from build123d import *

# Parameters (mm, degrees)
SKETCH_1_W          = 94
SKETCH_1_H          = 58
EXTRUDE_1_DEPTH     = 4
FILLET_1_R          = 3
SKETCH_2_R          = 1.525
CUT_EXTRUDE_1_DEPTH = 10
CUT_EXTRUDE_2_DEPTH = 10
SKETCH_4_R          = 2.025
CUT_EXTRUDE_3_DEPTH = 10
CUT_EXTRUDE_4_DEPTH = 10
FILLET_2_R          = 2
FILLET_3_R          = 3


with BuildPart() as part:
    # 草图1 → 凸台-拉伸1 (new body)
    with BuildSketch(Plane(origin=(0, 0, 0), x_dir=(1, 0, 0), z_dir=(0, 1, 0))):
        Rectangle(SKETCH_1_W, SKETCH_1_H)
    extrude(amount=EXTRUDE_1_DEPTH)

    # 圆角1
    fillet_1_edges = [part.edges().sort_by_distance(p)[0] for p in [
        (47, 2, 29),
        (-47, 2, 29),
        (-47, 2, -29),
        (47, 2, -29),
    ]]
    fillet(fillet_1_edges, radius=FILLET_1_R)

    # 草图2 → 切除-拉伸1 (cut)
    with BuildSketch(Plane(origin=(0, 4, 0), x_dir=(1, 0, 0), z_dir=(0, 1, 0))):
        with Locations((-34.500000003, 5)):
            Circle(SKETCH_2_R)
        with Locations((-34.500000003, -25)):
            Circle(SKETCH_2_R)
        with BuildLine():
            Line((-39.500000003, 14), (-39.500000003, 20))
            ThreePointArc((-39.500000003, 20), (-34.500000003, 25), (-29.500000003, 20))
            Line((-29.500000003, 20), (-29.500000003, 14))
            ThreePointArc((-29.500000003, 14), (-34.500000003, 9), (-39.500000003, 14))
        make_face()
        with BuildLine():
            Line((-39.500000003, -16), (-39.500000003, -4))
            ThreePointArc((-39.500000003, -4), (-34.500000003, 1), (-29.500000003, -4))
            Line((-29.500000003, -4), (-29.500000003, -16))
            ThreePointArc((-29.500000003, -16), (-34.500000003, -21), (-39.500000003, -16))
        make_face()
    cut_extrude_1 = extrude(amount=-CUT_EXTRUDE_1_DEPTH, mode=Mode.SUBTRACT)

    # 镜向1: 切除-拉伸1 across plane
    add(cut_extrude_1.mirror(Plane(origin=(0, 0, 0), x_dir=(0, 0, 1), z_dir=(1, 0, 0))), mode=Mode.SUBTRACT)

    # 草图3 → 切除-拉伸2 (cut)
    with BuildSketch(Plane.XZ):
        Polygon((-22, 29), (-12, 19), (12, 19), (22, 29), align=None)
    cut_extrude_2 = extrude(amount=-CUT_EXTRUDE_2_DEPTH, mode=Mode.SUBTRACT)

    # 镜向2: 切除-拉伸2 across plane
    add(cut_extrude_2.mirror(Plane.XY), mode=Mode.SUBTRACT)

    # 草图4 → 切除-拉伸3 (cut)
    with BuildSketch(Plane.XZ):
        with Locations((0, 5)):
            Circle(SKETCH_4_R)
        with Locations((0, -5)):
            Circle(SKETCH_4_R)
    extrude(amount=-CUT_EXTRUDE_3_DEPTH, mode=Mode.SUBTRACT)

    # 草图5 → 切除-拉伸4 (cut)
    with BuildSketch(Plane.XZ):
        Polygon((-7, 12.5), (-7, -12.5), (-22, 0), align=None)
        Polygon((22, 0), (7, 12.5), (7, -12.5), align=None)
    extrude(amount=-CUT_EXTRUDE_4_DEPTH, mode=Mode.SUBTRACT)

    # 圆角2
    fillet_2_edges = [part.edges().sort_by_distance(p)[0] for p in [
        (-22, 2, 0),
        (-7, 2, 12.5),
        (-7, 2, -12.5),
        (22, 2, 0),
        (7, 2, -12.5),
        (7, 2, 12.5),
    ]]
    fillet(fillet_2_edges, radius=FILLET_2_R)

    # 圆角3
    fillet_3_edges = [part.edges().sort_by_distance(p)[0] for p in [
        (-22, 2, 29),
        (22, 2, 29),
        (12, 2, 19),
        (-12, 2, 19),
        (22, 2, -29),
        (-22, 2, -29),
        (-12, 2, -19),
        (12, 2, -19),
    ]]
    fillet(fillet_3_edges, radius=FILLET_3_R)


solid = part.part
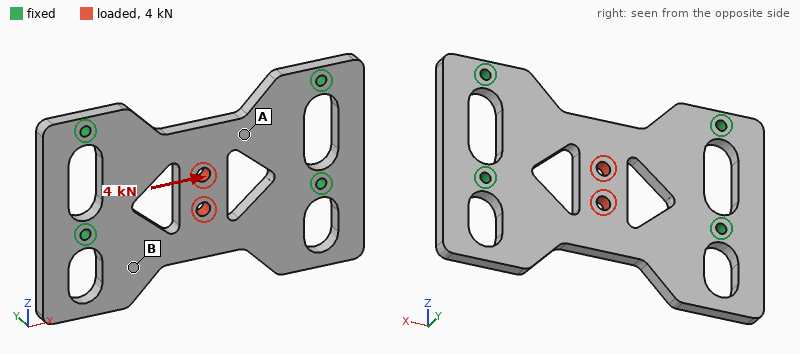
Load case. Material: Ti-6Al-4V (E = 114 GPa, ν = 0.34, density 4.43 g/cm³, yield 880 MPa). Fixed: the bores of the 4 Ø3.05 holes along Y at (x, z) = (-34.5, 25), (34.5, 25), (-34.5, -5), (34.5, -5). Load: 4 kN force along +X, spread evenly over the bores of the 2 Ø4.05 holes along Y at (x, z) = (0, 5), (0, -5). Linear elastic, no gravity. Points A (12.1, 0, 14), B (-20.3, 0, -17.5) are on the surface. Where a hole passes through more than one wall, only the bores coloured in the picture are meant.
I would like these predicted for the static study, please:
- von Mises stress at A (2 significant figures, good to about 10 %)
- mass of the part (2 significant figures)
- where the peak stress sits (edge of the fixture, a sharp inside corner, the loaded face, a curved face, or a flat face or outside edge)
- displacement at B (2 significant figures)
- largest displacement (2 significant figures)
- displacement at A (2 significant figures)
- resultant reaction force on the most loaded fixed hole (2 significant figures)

43 MPa
65 g
a curved face
8.1 µm
23 µm
5.7 µm
1.1 kN
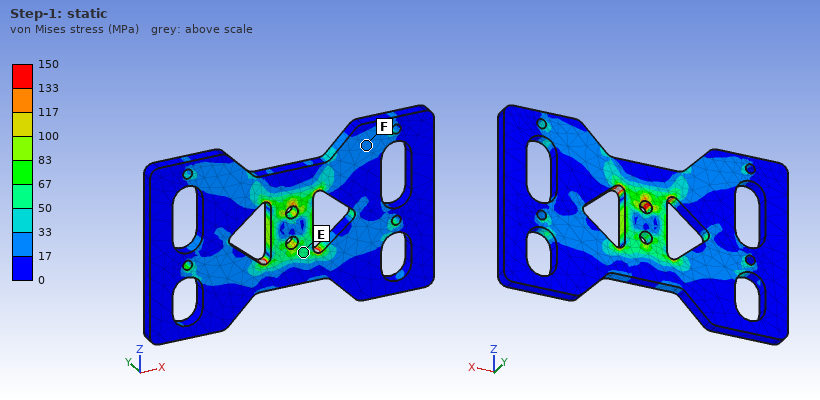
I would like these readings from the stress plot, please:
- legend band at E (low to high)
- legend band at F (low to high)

50 to 67 MPa
17 to 33 MPa
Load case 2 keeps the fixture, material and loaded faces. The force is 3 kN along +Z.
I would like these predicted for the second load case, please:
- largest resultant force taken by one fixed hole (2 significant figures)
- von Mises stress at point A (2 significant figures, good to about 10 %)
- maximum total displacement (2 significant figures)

1.1 kN
42 MPa
22 µm
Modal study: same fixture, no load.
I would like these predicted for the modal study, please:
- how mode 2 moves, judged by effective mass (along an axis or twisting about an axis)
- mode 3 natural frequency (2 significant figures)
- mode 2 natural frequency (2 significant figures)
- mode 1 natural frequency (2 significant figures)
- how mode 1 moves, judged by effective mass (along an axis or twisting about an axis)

twisting about X
4900 Hz
4300 Hz
3300 Hz
along Y
